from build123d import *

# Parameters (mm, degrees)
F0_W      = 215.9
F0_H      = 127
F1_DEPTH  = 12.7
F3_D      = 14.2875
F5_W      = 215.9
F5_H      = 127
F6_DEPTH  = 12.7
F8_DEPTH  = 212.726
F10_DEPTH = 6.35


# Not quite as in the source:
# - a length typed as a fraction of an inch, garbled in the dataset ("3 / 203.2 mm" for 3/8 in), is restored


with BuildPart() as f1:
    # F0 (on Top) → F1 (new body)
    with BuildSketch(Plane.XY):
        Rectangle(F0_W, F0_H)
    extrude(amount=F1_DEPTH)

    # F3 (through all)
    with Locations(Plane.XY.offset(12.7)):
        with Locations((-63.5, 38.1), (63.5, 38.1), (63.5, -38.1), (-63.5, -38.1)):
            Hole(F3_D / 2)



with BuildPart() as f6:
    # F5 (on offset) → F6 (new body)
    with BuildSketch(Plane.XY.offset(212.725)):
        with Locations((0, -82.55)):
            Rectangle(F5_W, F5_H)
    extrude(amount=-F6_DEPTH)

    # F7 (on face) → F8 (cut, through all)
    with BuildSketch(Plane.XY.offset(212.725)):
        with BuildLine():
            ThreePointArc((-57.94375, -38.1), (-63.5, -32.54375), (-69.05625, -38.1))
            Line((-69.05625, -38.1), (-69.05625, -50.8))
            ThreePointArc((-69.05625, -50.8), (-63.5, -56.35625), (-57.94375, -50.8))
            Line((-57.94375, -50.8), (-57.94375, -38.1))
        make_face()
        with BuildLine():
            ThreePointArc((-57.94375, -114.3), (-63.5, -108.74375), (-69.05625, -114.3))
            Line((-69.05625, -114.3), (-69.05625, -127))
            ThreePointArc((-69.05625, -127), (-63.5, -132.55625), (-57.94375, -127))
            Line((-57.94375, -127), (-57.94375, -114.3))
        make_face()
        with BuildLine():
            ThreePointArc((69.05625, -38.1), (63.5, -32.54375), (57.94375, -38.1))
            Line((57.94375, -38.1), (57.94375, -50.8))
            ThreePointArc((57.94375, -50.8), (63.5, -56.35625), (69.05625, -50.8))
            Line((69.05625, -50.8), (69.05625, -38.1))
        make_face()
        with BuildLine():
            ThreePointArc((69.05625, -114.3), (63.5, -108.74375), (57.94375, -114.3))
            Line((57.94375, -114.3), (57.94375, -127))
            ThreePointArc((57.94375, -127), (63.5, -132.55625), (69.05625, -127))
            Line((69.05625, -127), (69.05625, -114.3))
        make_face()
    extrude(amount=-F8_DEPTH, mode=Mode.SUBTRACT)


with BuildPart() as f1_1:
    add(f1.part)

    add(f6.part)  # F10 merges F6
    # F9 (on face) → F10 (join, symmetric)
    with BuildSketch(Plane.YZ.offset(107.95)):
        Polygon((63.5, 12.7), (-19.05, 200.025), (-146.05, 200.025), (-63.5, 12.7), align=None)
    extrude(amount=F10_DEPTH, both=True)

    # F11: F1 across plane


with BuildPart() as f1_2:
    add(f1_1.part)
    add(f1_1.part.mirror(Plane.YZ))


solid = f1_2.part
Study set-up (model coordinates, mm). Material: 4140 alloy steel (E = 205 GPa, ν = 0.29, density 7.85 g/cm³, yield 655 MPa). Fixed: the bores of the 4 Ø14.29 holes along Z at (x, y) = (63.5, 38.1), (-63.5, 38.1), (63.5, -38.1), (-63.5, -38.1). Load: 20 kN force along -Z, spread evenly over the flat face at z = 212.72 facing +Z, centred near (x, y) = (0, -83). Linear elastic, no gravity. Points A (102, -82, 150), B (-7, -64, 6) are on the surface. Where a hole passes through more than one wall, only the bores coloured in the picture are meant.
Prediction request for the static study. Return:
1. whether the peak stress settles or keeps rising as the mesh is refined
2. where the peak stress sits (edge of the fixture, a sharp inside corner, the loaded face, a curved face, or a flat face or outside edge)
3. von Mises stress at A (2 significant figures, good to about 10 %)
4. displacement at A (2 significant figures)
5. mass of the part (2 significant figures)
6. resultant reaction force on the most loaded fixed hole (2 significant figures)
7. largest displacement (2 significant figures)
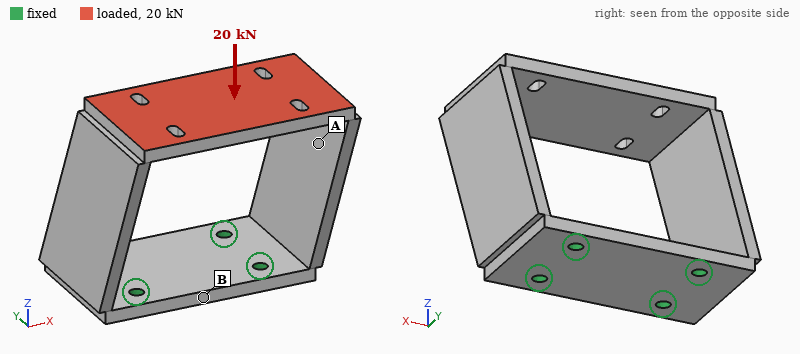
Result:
keeps rising
edge of the fixture
57 MPa
0.38 mm
10 kg
14 kN
0.83 mm
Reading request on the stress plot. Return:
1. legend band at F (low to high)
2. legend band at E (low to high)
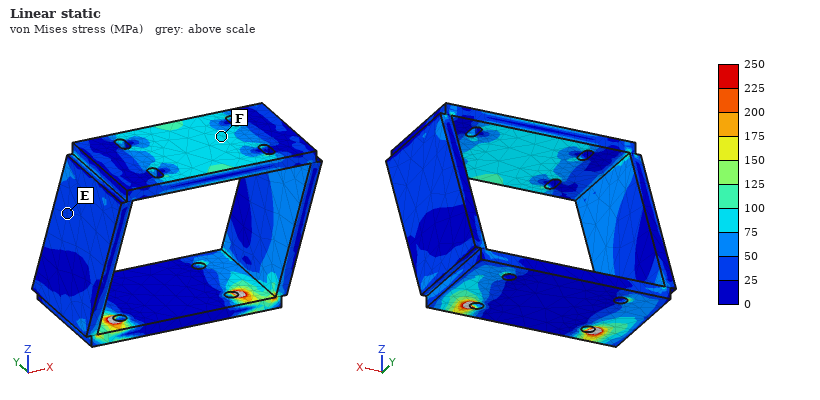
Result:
75 to 100 MPa
25 to 50 MPa
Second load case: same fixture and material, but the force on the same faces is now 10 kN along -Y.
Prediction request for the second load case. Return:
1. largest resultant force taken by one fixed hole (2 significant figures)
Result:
12 kN
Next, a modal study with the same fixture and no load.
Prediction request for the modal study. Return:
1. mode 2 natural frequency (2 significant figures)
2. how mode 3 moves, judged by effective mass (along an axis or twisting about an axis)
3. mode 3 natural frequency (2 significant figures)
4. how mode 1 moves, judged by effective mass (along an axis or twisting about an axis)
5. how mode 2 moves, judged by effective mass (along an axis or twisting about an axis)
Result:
330 Hz
twisting about Z
510 Hz
along X
along Y
